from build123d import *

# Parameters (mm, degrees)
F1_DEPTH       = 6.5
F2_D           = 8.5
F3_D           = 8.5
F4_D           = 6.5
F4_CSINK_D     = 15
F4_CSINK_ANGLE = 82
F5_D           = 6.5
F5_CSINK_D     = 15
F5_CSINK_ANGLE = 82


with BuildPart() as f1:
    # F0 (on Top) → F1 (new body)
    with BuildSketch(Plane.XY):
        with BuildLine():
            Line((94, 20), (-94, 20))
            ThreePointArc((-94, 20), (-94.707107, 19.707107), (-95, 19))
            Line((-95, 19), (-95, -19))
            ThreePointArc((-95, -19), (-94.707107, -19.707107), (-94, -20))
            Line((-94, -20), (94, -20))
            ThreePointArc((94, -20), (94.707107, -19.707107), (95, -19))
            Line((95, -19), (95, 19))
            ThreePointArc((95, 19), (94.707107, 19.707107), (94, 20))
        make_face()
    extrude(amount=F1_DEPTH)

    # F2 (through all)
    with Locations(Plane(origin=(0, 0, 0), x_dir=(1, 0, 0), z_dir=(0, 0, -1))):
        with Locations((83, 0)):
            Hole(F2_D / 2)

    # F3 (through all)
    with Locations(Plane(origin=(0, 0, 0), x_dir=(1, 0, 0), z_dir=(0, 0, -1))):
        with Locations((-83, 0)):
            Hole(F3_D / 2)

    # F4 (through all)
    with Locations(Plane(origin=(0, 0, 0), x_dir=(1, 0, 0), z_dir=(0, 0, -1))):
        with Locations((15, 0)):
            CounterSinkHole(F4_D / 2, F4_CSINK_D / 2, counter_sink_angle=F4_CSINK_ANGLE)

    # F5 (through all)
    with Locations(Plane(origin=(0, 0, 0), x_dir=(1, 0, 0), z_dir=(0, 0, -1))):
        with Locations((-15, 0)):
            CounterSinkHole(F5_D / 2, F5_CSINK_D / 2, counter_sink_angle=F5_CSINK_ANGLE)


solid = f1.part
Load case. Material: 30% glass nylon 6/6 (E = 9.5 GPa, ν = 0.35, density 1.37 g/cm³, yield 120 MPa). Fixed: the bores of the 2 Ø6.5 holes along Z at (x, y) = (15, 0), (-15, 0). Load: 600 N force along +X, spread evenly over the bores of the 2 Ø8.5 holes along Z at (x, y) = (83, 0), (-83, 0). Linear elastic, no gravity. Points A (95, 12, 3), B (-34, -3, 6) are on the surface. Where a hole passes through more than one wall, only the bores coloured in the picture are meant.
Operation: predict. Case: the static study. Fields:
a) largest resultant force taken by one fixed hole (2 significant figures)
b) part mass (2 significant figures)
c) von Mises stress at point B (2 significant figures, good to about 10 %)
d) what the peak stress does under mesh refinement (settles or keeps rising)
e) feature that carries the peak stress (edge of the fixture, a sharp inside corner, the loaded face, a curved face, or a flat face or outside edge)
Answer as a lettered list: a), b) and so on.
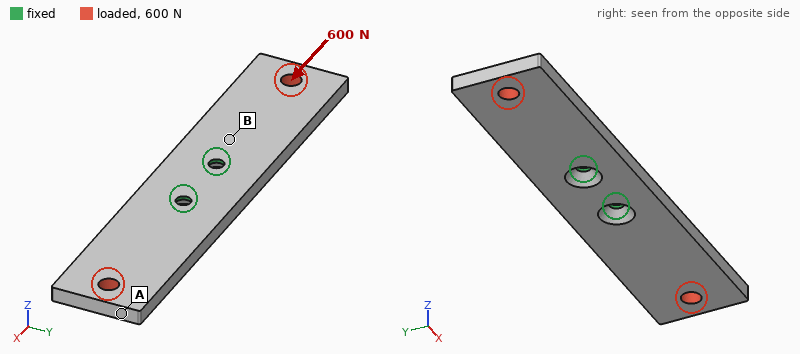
a) 300 N
b) 65 g
c) 1.5 MPa
d) keeps rising
e) edge of the fixture
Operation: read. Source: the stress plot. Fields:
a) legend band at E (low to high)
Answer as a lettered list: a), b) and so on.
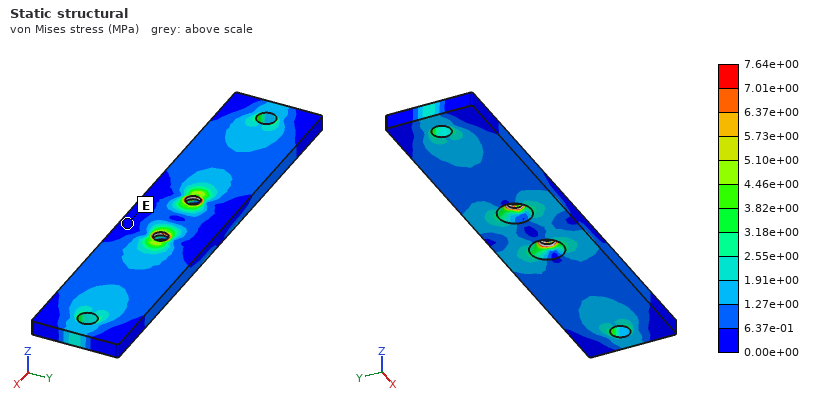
a) 0.00e+00 to 6.37e-01 MPa
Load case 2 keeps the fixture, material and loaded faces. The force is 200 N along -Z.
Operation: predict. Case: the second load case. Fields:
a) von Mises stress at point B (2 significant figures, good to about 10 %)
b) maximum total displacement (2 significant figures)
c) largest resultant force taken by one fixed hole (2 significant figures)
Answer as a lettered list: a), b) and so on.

a) 18 MPa
b) 2.0 mm
c) 880 N
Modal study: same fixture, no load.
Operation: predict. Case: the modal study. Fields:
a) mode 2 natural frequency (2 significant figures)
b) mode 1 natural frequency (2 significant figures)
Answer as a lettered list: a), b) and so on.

a) 380 Hz
b) 370 Hz
